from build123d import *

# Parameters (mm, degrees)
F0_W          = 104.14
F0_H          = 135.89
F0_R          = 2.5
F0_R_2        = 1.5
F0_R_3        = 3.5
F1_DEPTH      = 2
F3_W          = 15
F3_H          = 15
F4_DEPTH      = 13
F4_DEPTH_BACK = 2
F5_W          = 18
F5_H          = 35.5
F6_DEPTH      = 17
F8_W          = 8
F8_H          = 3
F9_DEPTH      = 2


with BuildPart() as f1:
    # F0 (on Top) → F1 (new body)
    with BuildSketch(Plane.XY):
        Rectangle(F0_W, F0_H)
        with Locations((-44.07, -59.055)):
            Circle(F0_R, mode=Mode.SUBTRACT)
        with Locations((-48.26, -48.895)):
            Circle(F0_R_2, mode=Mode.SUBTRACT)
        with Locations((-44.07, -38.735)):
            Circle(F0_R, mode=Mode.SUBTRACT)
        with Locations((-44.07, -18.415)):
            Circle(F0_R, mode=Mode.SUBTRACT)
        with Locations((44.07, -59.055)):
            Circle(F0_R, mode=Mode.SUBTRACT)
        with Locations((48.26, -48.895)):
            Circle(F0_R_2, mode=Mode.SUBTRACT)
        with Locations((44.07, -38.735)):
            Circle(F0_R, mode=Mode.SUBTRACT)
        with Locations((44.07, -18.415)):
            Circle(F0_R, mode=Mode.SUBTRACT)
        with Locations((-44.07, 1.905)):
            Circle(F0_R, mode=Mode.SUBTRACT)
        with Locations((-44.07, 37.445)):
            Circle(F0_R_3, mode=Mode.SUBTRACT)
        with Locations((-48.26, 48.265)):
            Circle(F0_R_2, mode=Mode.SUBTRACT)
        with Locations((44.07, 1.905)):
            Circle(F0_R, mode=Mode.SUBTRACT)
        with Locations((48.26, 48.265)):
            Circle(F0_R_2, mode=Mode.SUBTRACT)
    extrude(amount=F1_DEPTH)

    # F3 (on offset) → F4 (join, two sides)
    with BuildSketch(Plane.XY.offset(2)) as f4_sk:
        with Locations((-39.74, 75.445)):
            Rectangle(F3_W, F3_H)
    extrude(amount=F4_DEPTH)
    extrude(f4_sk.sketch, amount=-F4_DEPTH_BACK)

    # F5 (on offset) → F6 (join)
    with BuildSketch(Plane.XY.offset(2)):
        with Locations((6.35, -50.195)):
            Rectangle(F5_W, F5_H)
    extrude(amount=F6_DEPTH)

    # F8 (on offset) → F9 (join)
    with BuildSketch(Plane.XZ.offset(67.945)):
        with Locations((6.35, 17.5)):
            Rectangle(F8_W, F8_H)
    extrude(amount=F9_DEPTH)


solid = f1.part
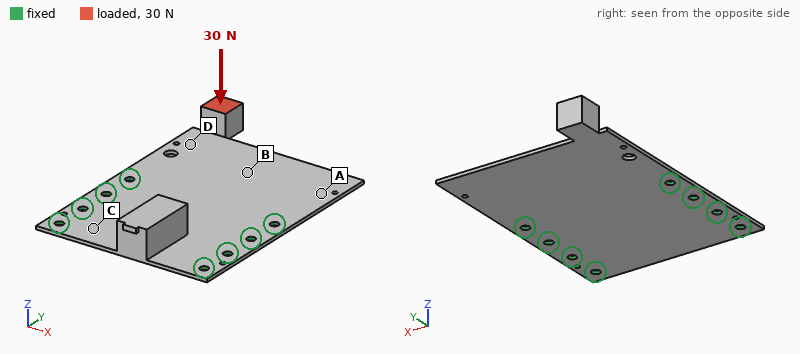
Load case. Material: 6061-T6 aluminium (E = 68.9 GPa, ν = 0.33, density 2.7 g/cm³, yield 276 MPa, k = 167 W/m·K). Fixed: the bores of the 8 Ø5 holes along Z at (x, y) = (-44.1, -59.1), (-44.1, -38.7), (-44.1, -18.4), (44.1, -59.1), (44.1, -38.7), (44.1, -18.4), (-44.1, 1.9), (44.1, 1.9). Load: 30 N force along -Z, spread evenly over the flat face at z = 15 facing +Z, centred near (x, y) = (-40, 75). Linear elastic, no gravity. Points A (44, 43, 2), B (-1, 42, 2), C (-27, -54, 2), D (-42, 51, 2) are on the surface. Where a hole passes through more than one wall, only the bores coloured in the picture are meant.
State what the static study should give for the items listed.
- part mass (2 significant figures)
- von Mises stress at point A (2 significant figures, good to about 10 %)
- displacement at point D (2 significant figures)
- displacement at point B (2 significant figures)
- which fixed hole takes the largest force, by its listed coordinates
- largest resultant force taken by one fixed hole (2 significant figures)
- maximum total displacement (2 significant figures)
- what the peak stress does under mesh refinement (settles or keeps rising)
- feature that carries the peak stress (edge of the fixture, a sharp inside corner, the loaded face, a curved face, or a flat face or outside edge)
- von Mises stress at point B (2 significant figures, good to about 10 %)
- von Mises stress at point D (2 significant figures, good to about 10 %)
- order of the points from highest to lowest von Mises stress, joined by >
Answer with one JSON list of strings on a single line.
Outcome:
["110 g", "11 MPa", "0.73 mm", "0.40 mm", "(-44.1, 1.9)", "52 N", "1.7 mm", "keeps rising", "edge of the fixture", "20 MPa", "26 MPa", "D > B > A > C"]
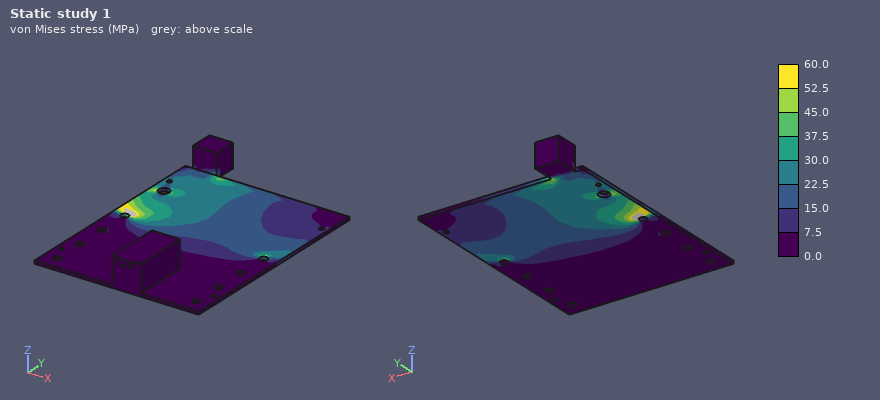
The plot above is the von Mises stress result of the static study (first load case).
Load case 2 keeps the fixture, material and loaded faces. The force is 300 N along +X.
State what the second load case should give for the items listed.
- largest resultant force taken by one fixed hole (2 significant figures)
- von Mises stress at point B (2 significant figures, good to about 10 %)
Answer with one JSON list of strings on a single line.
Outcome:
["250 N", "43 MPa"]
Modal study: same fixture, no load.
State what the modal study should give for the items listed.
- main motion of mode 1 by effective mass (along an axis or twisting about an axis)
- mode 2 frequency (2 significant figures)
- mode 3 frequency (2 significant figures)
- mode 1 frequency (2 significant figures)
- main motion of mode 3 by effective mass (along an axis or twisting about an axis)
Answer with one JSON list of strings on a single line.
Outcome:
["along Z", "500 Hz", "890 Hz", "200 Hz", "along Z"]
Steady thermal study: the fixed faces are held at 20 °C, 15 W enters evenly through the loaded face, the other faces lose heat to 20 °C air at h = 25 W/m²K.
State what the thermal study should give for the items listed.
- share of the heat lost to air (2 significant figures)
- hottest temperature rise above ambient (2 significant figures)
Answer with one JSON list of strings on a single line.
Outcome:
["44 %", "65 K"]
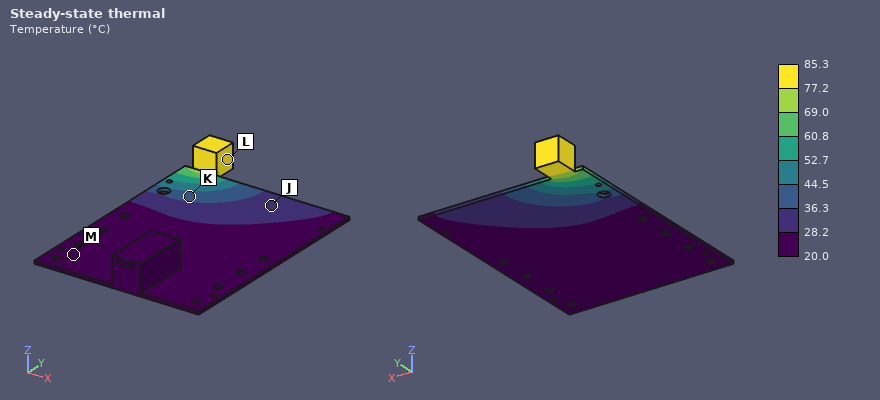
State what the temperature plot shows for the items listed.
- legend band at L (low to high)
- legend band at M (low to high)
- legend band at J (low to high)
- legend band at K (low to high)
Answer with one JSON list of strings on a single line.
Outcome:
["77.2 to 85.3 °C", "20.0 to 28.2 °C", "28.2 to 36.3 °C", "36.3 to 44.5 °C"]
